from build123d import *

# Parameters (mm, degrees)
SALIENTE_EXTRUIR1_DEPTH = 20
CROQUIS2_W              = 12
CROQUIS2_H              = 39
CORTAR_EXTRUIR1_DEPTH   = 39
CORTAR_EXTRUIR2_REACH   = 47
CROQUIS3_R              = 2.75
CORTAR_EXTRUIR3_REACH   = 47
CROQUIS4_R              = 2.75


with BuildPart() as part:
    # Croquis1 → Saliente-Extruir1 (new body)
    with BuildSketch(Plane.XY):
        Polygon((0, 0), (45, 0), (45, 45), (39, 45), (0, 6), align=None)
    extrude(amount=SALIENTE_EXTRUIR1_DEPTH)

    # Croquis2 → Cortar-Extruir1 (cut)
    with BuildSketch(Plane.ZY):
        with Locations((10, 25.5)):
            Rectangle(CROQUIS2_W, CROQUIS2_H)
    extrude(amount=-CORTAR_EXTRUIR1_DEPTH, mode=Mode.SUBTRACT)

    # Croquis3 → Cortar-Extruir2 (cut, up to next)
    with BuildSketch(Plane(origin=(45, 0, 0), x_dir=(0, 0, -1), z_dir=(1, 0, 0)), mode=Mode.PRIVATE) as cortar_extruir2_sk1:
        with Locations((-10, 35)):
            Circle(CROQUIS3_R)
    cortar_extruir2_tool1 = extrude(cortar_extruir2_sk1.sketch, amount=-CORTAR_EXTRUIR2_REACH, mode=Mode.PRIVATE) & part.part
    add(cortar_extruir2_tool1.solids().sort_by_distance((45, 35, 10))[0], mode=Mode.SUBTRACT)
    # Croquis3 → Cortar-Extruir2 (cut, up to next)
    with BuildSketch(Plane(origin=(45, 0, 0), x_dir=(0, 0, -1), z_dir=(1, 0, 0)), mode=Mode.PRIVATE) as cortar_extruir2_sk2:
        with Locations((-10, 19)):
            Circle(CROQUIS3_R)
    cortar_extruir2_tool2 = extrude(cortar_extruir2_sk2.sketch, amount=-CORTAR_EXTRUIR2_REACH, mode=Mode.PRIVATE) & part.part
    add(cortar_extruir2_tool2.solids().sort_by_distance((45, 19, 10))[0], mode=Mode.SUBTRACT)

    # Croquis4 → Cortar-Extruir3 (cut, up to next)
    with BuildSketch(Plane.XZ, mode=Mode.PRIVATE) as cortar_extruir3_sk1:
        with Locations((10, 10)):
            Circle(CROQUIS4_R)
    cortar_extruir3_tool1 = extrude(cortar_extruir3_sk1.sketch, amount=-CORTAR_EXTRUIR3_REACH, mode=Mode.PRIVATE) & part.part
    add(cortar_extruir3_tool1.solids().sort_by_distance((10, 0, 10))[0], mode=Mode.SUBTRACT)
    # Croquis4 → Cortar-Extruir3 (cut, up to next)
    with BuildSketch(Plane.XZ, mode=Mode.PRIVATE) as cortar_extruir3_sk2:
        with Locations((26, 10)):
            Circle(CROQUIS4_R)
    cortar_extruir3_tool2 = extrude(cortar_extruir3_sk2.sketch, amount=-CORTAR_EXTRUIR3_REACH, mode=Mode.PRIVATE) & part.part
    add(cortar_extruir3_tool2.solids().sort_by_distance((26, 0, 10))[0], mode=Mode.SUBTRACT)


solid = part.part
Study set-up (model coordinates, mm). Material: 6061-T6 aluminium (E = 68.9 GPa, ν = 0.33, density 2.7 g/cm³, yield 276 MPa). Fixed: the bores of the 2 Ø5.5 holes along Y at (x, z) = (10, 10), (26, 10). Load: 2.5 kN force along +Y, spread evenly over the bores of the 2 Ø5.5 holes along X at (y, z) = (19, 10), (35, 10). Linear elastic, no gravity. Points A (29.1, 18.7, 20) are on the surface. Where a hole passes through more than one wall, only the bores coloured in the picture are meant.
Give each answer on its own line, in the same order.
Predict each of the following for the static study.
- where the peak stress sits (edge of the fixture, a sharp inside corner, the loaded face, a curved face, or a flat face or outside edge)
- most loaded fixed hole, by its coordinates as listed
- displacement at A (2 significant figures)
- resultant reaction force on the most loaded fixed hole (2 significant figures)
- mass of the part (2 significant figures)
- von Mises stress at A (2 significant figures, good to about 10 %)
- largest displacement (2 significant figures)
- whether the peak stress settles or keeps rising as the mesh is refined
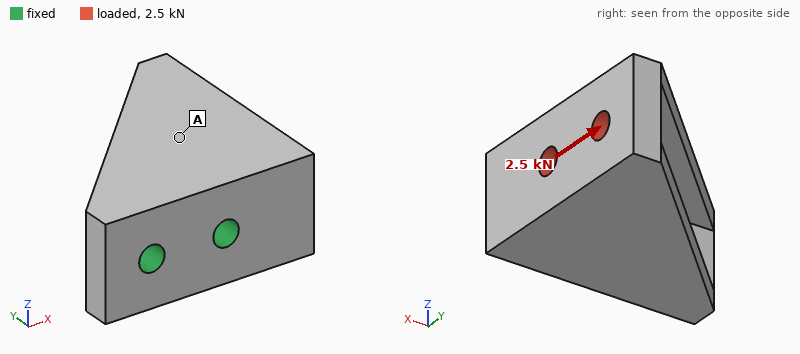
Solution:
edge of the fixture
(26, 10)
25 µm
3.9 kN
42 g
18 MPa
76 µm
keeps rising
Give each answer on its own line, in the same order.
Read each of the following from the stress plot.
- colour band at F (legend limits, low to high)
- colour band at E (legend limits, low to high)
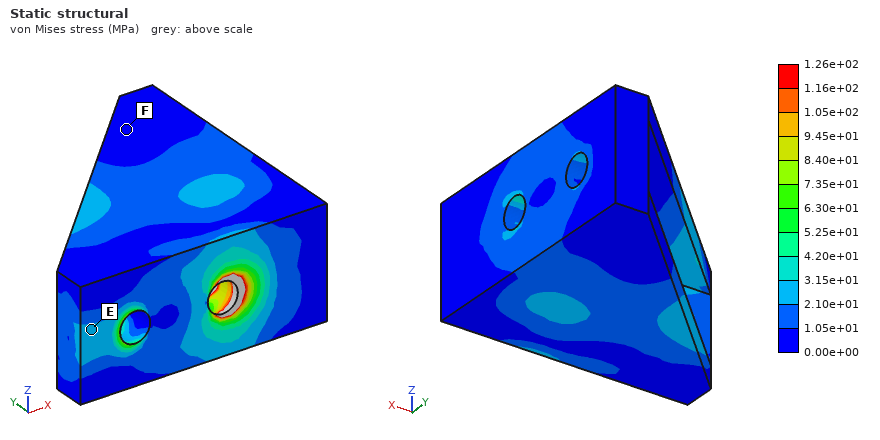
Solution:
0.00e+00 to 1.05e+01 MPa
2.10e+01 to 3.15e+01 MPa
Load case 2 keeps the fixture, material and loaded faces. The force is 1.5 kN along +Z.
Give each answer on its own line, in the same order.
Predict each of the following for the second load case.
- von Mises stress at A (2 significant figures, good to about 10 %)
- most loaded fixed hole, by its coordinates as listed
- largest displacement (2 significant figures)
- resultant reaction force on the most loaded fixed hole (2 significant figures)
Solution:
22 MPa
(26, 10)
0.23 mm
2.3 kN
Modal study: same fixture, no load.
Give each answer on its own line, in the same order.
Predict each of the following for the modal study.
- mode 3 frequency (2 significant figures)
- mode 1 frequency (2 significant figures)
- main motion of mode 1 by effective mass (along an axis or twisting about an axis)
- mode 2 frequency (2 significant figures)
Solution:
12 kHz
3500 Hz
along Z
6500 Hz
